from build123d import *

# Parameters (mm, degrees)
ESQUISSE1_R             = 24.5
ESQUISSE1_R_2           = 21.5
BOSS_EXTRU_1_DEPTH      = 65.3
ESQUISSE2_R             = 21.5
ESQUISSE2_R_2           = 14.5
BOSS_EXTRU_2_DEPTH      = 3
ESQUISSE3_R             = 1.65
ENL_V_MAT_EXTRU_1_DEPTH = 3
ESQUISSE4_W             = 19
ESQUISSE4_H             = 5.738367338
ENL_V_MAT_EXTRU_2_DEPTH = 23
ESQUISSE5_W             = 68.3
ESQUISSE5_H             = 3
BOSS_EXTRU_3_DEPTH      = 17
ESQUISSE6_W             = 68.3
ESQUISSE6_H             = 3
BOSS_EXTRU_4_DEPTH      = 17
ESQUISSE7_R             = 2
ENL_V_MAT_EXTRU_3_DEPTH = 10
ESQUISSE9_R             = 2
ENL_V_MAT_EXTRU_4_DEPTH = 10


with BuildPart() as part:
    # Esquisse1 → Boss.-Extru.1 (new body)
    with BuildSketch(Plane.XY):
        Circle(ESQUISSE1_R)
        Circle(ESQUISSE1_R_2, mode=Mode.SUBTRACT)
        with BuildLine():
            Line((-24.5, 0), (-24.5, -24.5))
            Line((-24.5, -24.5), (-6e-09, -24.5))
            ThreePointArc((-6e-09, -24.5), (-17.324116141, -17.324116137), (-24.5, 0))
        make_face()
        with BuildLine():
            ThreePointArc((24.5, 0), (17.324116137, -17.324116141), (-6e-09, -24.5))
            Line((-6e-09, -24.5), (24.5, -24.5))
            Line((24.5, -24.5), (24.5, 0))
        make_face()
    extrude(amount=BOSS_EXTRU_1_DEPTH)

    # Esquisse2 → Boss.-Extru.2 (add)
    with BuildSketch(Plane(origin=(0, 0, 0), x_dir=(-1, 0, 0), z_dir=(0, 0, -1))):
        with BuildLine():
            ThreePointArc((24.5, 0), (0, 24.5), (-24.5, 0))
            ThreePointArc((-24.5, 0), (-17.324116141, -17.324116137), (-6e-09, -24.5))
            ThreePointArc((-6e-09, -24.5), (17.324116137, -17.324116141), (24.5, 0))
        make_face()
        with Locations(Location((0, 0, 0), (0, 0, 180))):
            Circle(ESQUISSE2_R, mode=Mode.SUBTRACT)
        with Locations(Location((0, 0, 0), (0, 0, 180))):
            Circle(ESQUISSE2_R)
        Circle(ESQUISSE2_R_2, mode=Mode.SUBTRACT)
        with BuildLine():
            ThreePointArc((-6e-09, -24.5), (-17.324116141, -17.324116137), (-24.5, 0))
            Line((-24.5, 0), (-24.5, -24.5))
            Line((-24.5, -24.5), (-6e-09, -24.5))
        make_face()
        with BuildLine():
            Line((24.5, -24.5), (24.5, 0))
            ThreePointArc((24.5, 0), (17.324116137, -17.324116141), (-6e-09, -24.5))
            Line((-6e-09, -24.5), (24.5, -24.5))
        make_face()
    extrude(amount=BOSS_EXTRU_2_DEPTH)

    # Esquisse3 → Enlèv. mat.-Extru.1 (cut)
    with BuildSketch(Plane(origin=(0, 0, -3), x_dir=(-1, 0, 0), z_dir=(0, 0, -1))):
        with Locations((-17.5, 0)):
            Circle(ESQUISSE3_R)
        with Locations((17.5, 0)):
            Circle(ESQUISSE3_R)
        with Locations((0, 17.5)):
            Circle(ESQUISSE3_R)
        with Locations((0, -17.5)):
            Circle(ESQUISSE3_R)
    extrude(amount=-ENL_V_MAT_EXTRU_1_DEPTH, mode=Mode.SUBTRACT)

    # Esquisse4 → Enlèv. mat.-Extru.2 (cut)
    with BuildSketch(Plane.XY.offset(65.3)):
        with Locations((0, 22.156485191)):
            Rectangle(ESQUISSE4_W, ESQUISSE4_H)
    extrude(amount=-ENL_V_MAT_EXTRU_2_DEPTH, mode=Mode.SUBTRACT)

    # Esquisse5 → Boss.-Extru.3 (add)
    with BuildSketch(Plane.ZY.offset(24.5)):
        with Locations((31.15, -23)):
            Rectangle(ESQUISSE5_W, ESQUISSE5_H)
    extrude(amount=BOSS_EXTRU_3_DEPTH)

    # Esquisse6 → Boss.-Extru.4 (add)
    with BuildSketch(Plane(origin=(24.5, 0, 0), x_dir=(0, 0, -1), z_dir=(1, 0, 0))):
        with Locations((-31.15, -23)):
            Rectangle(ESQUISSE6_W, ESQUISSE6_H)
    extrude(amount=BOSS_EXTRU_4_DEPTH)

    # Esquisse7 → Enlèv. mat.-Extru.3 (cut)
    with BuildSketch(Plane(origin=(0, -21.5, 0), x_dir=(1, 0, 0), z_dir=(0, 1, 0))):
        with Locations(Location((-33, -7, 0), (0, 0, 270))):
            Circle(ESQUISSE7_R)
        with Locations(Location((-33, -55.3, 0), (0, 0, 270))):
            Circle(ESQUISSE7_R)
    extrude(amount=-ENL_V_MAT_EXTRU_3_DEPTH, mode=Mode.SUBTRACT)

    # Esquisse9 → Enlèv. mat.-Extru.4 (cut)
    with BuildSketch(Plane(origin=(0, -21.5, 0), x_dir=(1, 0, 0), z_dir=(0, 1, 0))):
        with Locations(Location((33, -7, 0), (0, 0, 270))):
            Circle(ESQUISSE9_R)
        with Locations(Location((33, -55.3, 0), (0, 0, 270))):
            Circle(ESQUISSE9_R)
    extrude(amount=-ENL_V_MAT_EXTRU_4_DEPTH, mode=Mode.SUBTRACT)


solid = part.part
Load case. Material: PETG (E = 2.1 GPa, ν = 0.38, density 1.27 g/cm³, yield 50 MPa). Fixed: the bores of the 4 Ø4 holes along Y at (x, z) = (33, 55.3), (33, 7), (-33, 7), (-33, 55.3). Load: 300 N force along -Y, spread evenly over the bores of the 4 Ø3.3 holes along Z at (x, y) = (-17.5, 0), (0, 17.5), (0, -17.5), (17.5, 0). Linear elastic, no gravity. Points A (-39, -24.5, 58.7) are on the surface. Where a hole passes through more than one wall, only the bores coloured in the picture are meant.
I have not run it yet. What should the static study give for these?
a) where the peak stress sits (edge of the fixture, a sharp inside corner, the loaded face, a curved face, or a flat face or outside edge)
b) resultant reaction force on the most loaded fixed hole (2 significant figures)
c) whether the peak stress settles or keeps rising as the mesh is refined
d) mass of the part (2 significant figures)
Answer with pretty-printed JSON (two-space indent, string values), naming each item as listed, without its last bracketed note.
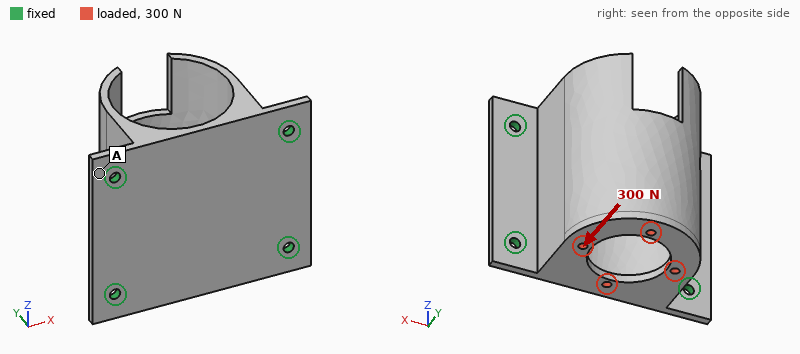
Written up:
{
  "where the peak stress sits": "edge of the fixture",
  "resultant reaction force on the most loaded fixed hole": "190 N",
  "whether the peak stress settles or keeps rising as the mesh is refined": "keeps rising",
  "mass of the part": "70 g"
}
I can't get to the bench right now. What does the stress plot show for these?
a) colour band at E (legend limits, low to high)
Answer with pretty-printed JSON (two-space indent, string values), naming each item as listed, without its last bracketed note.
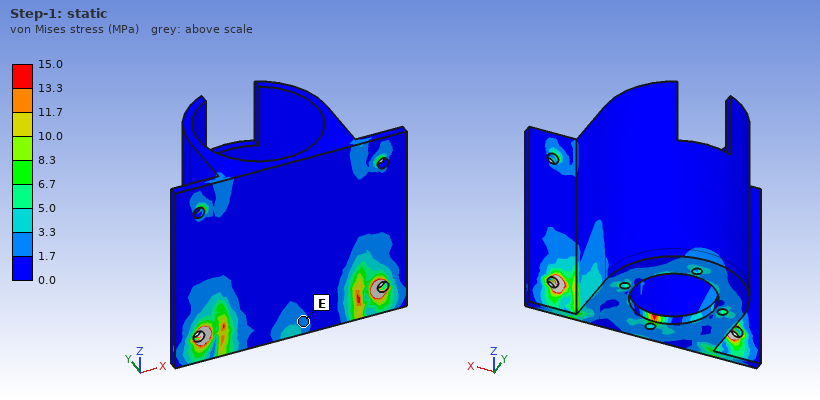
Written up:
{
  "colour band at E": "1.7 to 3.3 MPa"
}
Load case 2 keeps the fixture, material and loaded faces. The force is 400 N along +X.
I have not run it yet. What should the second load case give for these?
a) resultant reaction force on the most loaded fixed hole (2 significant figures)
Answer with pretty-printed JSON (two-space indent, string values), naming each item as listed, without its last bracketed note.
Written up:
{
  "resultant reaction force on the most loaded fixed hole": "190 N"
}
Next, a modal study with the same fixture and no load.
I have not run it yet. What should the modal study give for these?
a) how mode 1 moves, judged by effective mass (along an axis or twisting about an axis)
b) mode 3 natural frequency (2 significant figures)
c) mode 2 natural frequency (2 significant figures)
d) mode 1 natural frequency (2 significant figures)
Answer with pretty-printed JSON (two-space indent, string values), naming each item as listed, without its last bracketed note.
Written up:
{
  "how mode 1 moves, judged by effective mass": "along X",
  "mode 3 natural frequency": "930 Hz",
  "mode 2 natural frequency": "880 Hz",
  "mode 1 natural frequency": "790 Hz"
}
